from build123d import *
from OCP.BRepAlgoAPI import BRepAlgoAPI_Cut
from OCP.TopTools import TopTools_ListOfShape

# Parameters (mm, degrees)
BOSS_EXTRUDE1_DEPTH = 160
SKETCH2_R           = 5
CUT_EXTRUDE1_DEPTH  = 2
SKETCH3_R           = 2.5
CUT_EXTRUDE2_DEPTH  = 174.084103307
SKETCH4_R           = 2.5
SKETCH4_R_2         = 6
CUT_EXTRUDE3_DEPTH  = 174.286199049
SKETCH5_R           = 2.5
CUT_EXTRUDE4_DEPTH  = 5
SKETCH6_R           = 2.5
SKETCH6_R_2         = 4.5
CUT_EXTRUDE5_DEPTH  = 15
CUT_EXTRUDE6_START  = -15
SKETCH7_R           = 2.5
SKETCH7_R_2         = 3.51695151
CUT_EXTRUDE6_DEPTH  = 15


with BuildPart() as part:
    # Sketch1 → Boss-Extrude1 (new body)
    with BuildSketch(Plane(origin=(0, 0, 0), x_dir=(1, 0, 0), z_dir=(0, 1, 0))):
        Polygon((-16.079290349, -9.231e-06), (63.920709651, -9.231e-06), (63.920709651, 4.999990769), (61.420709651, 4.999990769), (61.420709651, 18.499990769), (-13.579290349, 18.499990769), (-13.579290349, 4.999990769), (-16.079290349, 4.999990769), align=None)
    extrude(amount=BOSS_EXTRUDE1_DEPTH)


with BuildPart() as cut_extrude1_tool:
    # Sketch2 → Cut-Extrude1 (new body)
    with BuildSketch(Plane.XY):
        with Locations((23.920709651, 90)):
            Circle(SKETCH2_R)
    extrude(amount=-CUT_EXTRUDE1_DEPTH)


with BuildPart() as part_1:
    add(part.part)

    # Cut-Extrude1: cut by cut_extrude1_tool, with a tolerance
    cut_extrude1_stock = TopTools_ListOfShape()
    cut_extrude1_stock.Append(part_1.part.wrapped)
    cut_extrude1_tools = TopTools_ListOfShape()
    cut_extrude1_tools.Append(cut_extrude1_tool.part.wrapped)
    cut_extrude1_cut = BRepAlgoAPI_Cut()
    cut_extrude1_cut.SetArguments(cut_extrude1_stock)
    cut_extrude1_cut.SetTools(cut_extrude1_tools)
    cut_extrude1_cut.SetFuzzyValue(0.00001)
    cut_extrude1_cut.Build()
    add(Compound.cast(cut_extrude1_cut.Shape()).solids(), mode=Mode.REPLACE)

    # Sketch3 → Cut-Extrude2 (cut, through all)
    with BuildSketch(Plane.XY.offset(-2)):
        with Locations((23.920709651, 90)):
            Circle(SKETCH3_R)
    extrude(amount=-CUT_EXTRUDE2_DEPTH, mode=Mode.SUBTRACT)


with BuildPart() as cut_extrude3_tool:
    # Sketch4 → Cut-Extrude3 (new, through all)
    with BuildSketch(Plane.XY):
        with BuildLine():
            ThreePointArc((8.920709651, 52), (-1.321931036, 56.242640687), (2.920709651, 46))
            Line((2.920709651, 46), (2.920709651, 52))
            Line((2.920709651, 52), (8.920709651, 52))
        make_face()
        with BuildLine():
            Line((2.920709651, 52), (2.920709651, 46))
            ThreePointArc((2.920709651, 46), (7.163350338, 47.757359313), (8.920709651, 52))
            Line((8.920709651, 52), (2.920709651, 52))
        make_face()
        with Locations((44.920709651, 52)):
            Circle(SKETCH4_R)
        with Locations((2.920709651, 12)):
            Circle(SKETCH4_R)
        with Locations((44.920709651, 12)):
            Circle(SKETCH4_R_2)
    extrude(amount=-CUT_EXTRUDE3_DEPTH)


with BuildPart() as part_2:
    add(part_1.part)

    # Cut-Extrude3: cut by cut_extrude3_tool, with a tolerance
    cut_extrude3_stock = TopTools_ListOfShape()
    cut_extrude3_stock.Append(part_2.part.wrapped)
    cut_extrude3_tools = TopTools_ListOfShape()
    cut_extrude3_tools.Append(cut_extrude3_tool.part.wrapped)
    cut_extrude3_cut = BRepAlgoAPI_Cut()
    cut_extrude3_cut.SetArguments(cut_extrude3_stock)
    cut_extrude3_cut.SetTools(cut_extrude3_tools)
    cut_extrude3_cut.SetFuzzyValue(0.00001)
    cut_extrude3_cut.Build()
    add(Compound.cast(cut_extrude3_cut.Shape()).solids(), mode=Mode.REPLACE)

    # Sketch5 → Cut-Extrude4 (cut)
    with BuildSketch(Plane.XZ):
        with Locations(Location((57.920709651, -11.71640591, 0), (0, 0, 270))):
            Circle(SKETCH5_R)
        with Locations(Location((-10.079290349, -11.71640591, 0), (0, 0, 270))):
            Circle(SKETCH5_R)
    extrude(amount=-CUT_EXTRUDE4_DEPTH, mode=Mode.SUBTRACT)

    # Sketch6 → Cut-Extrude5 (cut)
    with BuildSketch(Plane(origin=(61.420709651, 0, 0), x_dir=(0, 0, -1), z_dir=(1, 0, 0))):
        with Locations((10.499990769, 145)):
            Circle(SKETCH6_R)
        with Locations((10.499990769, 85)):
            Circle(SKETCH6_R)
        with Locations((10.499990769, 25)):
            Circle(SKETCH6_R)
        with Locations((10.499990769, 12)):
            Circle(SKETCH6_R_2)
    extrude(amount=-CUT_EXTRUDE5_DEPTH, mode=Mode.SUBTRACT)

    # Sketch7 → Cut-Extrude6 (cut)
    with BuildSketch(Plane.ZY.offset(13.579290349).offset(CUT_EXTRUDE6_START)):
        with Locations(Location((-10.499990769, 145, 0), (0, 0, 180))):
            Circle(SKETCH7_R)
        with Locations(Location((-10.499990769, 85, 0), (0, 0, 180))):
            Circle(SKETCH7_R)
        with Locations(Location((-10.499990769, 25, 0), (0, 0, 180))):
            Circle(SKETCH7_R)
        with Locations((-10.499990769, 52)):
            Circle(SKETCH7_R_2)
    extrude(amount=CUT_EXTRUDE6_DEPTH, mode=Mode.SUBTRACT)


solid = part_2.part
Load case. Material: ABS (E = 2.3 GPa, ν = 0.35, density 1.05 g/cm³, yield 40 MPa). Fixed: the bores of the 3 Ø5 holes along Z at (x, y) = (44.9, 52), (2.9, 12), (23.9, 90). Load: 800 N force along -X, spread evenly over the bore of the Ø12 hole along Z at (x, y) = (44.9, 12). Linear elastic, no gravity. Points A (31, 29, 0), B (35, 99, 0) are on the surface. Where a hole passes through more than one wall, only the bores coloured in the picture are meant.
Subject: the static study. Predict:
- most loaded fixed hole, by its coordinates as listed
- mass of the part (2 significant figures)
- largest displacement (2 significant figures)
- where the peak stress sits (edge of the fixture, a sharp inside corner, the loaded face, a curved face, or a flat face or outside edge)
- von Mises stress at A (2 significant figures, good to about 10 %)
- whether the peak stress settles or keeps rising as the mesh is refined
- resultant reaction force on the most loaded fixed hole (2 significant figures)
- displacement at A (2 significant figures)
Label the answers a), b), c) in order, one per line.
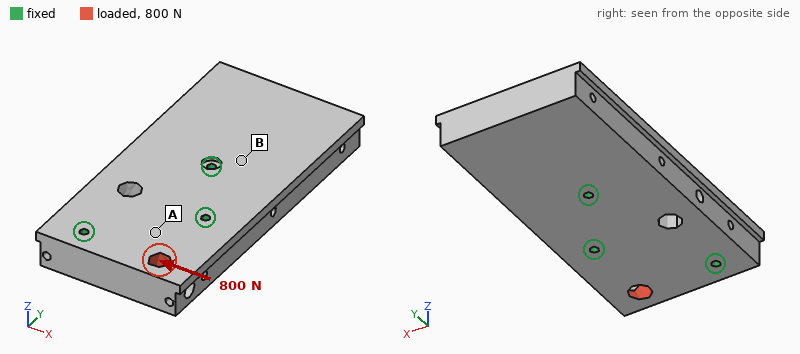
a) (2.9, 12)
b) 230 g
c) 40 µm
d) edge of the fixture
e) 0.68 MPa
f) keeps rising
g) 630 N
h) 12 µm
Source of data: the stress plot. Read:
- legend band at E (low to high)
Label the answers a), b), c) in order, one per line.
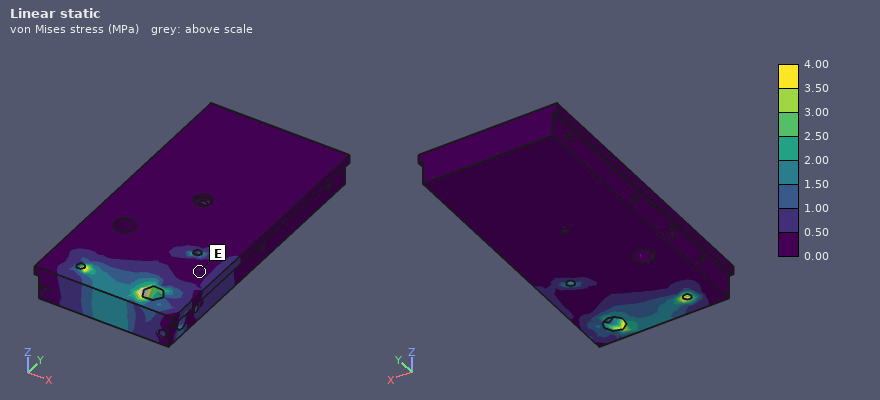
a) 0.00 to 0.50 MPa
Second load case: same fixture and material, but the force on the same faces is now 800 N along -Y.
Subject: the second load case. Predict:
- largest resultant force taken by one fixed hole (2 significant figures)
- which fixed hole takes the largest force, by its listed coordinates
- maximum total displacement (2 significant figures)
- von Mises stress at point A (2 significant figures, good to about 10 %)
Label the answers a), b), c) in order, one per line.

a) 550 N
b) (44.9, 52)
c) 44 µm
d) 0.95 MPa
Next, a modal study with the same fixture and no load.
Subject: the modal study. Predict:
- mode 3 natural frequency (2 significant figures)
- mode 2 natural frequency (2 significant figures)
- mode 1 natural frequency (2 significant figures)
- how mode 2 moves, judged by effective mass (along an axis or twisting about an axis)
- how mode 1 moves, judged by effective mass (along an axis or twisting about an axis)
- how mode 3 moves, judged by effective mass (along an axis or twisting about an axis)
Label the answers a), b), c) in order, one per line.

a) 1400 Hz
b) 1100 Hz
c) 680 Hz
d) twisting about Y
e) along Z
f) along X
